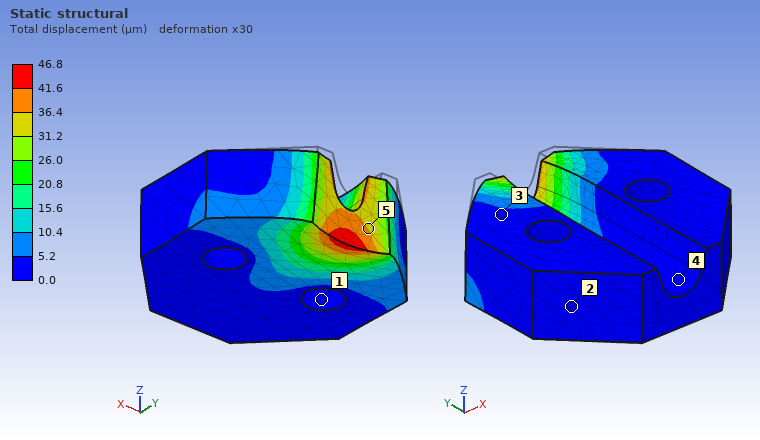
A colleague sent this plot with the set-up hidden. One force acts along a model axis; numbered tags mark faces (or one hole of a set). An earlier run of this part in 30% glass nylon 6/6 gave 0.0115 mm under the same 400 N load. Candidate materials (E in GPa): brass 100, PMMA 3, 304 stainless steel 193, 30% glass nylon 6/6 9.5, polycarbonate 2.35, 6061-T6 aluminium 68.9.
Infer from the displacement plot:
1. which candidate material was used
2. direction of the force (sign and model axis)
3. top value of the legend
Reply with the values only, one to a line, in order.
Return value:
polycarbonate
-Y
46.8 µm
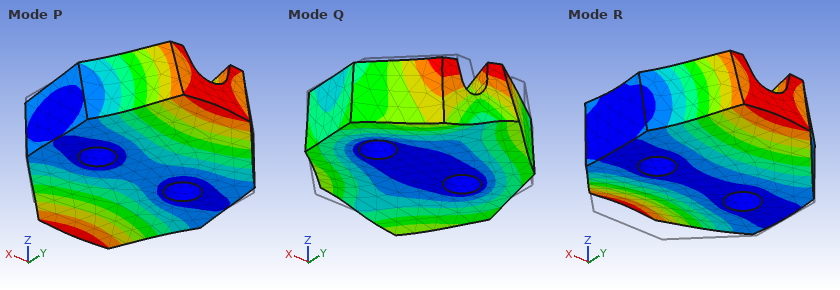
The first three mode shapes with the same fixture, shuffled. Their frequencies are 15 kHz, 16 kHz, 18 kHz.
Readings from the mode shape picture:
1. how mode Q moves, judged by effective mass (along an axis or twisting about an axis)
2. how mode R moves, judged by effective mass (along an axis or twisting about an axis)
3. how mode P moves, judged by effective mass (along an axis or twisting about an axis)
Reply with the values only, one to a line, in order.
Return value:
twisting about Z
along Z
twisting about X
